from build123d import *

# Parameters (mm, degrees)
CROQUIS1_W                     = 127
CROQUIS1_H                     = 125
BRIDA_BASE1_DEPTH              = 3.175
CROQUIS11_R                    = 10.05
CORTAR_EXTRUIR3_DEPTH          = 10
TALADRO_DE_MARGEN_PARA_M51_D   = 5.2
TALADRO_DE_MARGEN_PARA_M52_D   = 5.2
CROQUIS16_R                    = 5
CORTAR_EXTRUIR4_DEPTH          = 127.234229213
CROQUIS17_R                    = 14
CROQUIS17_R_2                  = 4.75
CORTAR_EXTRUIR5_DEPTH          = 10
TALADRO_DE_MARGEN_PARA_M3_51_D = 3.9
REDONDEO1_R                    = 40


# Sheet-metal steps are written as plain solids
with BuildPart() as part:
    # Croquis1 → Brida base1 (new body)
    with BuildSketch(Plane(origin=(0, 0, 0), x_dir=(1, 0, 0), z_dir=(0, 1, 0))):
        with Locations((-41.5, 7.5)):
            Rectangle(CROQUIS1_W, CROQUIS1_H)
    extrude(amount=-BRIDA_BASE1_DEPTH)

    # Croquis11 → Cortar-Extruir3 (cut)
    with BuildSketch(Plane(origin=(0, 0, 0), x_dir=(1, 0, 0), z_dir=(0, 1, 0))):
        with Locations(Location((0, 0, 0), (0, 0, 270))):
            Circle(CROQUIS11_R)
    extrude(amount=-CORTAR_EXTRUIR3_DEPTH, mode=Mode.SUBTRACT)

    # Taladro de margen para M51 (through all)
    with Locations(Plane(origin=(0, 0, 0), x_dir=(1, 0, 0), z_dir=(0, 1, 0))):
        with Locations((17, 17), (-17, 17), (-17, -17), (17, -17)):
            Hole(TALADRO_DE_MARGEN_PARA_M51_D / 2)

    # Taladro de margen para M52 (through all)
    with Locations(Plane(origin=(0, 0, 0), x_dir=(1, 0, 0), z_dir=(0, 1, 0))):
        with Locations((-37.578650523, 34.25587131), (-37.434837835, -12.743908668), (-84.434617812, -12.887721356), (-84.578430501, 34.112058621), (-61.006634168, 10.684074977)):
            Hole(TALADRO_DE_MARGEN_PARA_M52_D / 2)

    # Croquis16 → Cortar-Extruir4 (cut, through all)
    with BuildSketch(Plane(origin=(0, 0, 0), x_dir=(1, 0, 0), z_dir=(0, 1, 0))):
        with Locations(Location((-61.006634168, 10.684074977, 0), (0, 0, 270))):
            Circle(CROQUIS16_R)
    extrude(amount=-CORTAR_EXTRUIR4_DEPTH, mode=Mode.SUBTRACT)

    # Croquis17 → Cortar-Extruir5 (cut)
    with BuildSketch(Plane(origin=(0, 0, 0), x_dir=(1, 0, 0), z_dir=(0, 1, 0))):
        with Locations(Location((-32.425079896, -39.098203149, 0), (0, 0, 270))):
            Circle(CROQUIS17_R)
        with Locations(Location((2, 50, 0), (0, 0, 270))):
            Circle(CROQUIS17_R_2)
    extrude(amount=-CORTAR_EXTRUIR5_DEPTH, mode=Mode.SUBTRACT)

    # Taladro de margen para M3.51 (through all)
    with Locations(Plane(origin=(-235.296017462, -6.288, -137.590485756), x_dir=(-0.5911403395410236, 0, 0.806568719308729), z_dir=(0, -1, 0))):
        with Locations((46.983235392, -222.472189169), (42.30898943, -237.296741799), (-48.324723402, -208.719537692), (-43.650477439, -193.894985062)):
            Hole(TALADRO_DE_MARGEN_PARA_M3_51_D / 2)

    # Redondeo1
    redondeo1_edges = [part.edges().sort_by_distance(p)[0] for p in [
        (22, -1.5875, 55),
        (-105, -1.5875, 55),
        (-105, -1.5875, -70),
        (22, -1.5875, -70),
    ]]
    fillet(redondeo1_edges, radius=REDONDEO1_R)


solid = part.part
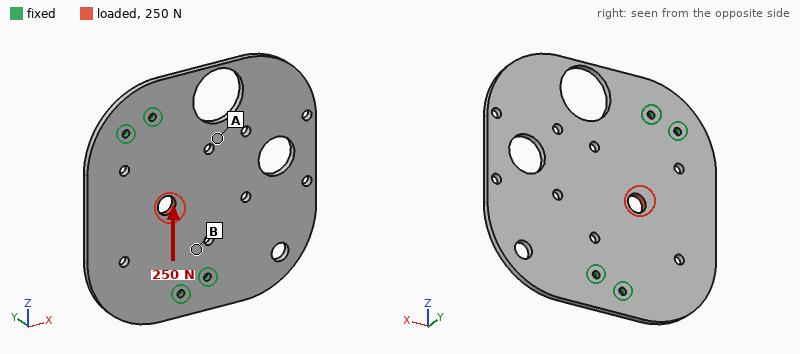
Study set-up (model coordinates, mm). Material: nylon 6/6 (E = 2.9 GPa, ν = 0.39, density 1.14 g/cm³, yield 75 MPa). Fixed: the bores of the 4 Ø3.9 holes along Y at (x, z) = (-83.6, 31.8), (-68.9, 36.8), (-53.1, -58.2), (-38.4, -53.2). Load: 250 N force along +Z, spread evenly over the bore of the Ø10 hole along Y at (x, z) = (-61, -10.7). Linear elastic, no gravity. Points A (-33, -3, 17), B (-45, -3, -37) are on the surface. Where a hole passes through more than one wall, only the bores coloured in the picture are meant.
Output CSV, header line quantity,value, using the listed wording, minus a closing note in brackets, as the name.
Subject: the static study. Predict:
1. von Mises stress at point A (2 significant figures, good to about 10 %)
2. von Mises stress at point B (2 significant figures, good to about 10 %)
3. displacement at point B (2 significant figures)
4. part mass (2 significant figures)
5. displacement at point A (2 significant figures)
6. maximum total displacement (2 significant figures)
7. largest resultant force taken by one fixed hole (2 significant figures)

quantity,value
von Mises stress at point A,0.30 MPa
von Mises stress at point B,1.1 MPa
displacement at point B,7.1 µm
part mass,48 g
displacement at point A,12 µm
maximum total displacement,24 µm
largest resultant force taken by one fixed hole,75 N
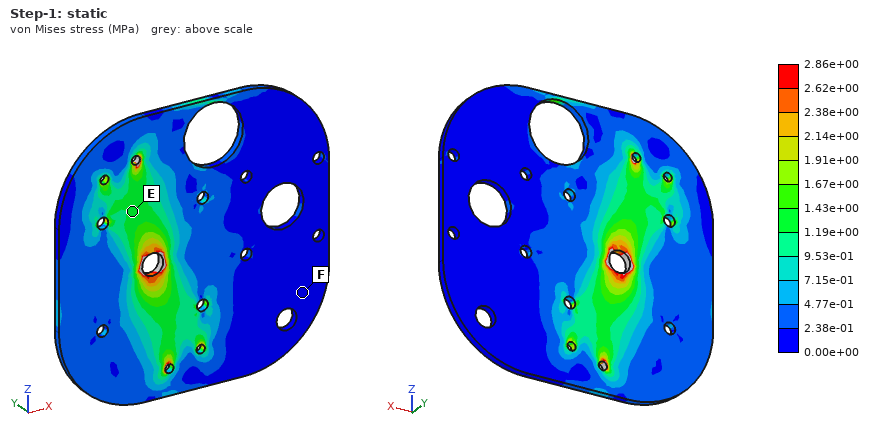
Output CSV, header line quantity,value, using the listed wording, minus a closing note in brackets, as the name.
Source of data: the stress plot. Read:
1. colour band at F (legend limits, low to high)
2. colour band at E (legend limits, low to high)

quantity,value
colour band at F,0.00e+00 to 2.38e-01 MPa
colour band at E,1.19e+00 to 1.43e+00 MPa
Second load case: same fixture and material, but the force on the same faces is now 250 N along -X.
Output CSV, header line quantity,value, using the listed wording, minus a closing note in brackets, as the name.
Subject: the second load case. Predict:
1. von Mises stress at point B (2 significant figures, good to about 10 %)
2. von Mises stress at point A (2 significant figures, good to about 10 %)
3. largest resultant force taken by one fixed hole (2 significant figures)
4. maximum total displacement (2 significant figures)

quantity,value
von Mises stress at point B,1.0 MPa
von Mises stress at point A,0.82 MPa
largest resultant force taken by one fixed hole,76 N
maximum total displacement,37 µm
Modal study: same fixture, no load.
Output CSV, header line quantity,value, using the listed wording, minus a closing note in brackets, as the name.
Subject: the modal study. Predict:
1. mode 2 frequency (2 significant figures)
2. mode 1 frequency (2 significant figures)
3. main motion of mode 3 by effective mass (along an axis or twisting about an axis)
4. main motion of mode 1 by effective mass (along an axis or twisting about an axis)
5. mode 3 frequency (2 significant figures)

quantity,value
mode 2 frequency,320 Hz
mode 1 frequency,140 Hz
main motion of mode 3 by effective mass,along Y
main motion of mode 1 by effective mass,along Y
mode 3 frequency,380 Hz
